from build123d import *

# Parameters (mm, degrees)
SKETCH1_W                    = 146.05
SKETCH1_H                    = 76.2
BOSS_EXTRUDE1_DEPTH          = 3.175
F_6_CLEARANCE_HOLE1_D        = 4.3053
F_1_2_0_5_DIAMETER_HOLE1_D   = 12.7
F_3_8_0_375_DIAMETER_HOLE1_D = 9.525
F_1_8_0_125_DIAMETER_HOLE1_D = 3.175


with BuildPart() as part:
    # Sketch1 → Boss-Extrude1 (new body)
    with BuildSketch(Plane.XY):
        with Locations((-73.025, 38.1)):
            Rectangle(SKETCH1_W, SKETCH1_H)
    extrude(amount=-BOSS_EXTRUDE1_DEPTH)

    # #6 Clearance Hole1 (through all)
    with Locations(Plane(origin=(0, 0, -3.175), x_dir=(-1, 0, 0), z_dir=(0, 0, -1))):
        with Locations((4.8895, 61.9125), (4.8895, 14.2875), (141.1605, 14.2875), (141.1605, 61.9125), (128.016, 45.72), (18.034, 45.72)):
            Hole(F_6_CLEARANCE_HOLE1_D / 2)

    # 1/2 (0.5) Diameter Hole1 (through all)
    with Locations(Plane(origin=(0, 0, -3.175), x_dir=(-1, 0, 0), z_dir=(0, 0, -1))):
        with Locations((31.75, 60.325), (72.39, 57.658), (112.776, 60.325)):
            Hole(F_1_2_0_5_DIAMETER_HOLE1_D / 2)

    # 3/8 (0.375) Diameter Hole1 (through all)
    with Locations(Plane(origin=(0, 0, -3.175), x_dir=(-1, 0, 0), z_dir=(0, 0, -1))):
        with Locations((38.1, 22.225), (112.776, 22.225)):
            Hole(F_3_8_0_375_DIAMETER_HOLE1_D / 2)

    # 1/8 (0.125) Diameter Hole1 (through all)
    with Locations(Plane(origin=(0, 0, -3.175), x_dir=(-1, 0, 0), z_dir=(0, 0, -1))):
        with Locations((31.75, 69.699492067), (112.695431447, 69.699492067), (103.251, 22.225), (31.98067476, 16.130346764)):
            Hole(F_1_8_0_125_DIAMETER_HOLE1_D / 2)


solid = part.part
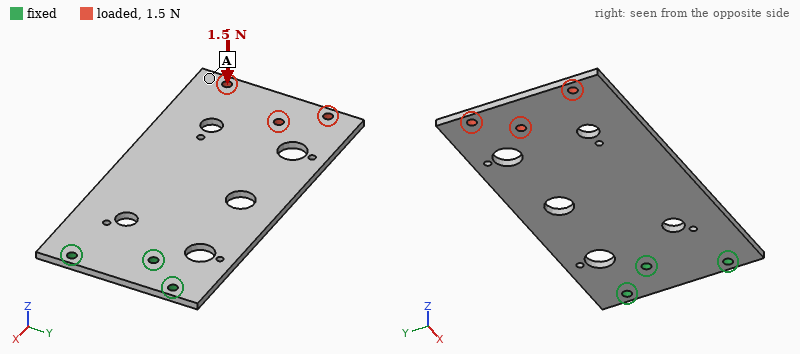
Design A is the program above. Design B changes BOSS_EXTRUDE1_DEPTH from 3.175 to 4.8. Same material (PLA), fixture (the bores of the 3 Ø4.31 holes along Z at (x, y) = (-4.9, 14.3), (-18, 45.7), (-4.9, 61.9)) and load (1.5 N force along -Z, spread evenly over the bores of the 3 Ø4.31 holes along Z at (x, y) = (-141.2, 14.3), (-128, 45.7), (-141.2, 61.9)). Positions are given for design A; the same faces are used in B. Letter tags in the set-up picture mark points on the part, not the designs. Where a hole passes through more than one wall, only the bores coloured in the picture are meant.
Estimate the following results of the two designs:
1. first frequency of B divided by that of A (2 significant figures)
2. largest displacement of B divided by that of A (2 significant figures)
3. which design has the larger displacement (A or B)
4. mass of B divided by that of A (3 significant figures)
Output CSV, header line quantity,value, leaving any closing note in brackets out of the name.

quantity,value
first frequency of B divided by that of A,1.5
largest displacement of B divided by that of A,0.30
which design has the larger displacement,A
mass of B divided by that of A,1.51
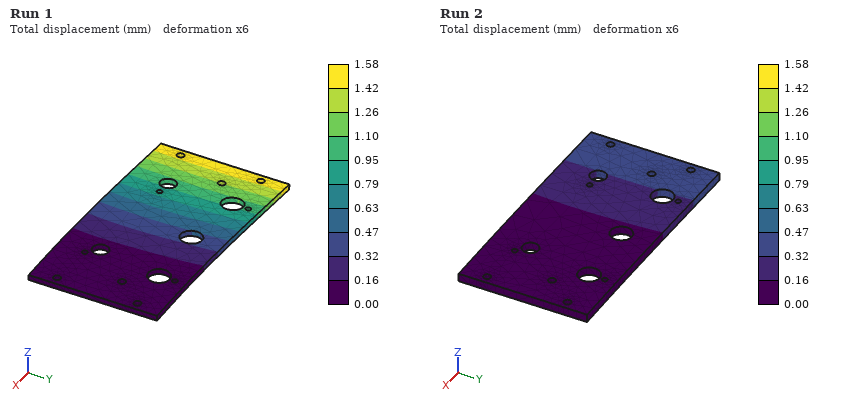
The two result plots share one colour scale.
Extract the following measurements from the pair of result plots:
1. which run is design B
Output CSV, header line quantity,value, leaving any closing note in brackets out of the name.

quantity,value
which run is design B,Run 2
